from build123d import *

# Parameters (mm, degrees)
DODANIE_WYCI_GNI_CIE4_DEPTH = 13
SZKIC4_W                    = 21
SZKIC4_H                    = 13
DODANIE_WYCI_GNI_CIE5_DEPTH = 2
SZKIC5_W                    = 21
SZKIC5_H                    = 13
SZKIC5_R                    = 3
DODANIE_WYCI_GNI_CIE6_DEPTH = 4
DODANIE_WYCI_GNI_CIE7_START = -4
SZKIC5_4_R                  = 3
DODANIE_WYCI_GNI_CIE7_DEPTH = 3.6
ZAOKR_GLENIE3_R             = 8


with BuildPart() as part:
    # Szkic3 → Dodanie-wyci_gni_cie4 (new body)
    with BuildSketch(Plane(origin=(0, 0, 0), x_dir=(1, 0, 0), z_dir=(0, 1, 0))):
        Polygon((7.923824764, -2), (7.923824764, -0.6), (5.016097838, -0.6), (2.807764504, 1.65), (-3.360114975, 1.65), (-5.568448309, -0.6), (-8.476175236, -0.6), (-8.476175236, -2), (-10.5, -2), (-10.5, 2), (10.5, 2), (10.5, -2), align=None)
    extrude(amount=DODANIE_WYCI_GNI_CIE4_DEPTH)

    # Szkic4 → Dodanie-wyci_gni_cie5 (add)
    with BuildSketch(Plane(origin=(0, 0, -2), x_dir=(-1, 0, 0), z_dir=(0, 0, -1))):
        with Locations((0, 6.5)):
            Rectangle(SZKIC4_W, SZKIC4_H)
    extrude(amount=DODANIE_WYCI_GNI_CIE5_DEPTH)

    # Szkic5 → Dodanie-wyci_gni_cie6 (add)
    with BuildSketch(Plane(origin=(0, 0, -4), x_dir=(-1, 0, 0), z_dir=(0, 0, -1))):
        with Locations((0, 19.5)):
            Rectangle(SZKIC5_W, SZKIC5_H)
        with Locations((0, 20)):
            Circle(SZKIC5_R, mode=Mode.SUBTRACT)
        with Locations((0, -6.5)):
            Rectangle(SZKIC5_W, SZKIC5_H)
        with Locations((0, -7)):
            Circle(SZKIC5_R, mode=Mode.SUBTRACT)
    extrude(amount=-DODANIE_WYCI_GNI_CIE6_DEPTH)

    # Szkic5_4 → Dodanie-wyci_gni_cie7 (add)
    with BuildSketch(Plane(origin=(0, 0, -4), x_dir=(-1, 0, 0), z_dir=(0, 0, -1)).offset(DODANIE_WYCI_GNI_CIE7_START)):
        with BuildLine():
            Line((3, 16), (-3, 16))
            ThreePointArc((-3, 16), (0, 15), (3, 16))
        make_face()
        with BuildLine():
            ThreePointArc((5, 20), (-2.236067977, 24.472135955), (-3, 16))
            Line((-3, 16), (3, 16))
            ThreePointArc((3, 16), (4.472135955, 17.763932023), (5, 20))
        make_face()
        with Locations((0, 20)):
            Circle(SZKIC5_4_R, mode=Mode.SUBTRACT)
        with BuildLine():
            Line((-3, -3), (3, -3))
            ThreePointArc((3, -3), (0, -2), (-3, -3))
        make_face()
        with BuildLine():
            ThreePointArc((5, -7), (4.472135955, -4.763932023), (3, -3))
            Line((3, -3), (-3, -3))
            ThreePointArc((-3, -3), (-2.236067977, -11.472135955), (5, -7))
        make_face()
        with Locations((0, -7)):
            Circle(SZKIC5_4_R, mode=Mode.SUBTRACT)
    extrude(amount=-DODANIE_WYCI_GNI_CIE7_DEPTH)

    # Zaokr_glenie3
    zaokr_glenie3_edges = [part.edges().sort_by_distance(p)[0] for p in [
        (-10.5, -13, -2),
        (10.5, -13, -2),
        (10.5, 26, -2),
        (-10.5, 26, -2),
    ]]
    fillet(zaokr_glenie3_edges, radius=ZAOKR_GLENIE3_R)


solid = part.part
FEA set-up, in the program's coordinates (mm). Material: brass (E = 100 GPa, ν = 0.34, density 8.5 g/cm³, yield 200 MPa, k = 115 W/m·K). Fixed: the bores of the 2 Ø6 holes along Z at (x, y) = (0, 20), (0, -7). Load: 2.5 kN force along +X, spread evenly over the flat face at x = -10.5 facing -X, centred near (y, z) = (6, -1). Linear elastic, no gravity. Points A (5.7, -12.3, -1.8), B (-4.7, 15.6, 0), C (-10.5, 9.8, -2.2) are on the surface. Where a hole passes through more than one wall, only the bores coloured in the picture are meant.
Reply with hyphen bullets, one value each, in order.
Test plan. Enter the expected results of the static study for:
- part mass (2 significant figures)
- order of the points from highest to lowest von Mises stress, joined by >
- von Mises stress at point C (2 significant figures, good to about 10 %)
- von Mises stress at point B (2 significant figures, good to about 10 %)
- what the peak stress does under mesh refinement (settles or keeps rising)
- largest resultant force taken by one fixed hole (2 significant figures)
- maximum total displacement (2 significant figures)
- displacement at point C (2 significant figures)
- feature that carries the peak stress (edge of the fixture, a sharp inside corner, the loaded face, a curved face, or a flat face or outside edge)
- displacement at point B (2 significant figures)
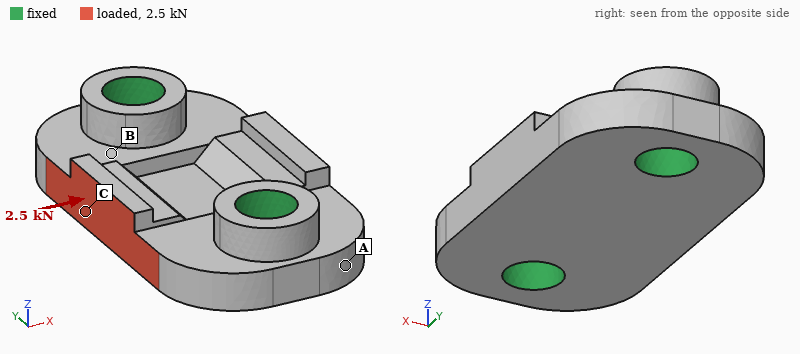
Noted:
- 27 g
- B > C > A
- 45 MPa
- 76 MPa
- keeps rising
- 1.3 kN
- 18 µm
- 11 µm
- a sharp inside corner
- 2.8 µm
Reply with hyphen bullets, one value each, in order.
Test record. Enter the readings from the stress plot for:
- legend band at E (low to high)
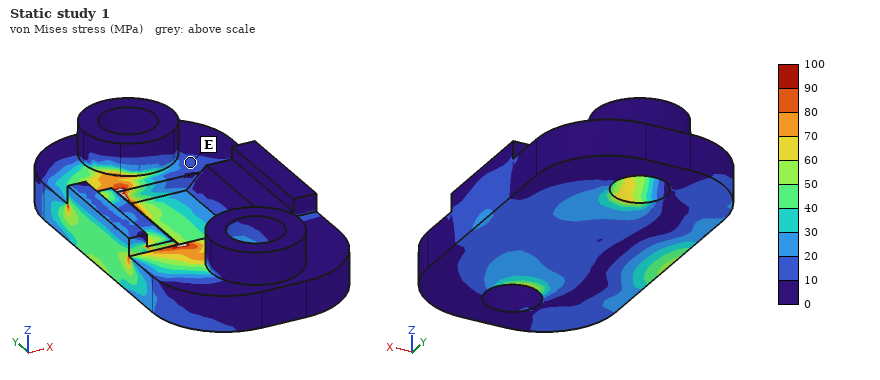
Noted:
- 10 to 20 MPa
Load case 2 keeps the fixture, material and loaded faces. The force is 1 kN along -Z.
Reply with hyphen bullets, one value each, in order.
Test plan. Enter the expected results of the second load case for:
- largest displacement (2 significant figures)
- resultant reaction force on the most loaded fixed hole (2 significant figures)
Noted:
- 36 µm
- 500 N
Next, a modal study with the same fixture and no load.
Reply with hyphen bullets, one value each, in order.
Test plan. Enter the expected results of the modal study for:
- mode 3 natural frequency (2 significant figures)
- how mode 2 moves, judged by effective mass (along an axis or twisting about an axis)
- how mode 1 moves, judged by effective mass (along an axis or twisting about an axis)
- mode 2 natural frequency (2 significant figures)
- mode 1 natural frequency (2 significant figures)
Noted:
- 34 kHz
- along Z
- twisting about Y
- 18 kHz
- 17 kHz
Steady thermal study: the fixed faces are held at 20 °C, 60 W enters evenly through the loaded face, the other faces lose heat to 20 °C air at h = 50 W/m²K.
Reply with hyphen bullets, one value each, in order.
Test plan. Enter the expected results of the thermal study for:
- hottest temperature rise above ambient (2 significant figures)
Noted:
- 66 K
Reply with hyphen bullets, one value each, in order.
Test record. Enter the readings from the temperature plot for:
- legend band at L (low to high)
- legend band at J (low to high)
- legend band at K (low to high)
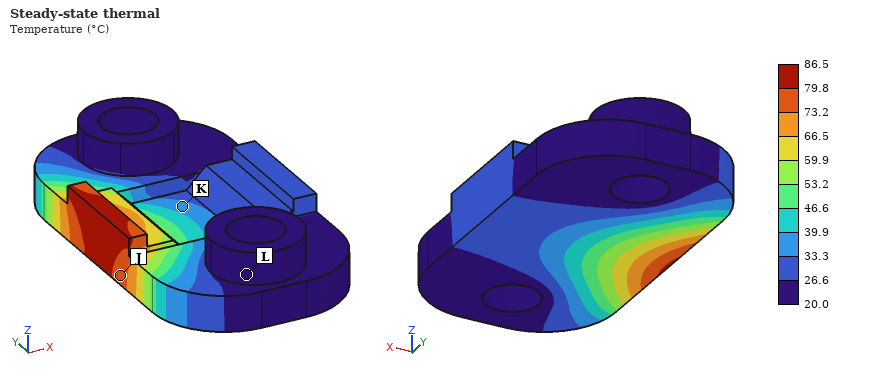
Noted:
- 20.0 to 26.6 °C
- 73.2 to 79.8 °C
- 33.3 to 39.9 °C
